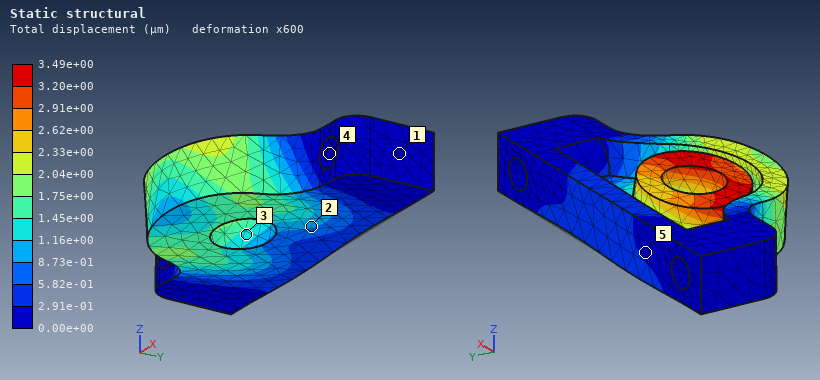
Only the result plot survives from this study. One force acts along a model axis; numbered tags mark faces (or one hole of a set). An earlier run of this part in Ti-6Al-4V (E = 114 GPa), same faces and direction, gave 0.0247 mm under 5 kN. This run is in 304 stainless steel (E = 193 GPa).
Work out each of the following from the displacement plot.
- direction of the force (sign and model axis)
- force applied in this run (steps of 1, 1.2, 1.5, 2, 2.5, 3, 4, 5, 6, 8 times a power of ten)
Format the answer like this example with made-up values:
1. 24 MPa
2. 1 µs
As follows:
1. -X
2. 1.2 kN
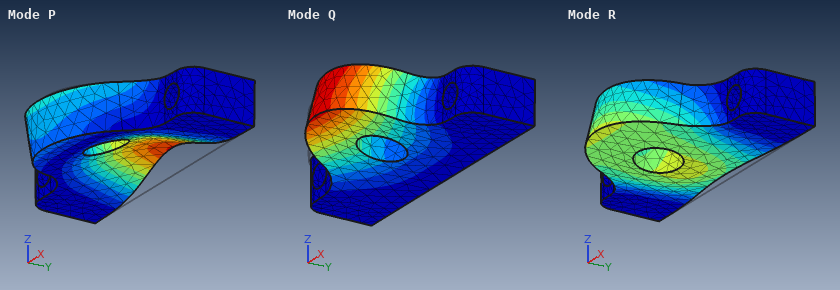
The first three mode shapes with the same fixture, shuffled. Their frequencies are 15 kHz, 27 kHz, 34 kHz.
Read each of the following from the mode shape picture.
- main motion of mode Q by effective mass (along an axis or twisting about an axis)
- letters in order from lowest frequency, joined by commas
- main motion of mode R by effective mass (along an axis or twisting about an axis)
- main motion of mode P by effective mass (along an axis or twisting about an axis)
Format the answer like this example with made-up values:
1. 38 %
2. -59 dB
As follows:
1. along Z
2. Q, P, R
3. along Y
4. along Z
